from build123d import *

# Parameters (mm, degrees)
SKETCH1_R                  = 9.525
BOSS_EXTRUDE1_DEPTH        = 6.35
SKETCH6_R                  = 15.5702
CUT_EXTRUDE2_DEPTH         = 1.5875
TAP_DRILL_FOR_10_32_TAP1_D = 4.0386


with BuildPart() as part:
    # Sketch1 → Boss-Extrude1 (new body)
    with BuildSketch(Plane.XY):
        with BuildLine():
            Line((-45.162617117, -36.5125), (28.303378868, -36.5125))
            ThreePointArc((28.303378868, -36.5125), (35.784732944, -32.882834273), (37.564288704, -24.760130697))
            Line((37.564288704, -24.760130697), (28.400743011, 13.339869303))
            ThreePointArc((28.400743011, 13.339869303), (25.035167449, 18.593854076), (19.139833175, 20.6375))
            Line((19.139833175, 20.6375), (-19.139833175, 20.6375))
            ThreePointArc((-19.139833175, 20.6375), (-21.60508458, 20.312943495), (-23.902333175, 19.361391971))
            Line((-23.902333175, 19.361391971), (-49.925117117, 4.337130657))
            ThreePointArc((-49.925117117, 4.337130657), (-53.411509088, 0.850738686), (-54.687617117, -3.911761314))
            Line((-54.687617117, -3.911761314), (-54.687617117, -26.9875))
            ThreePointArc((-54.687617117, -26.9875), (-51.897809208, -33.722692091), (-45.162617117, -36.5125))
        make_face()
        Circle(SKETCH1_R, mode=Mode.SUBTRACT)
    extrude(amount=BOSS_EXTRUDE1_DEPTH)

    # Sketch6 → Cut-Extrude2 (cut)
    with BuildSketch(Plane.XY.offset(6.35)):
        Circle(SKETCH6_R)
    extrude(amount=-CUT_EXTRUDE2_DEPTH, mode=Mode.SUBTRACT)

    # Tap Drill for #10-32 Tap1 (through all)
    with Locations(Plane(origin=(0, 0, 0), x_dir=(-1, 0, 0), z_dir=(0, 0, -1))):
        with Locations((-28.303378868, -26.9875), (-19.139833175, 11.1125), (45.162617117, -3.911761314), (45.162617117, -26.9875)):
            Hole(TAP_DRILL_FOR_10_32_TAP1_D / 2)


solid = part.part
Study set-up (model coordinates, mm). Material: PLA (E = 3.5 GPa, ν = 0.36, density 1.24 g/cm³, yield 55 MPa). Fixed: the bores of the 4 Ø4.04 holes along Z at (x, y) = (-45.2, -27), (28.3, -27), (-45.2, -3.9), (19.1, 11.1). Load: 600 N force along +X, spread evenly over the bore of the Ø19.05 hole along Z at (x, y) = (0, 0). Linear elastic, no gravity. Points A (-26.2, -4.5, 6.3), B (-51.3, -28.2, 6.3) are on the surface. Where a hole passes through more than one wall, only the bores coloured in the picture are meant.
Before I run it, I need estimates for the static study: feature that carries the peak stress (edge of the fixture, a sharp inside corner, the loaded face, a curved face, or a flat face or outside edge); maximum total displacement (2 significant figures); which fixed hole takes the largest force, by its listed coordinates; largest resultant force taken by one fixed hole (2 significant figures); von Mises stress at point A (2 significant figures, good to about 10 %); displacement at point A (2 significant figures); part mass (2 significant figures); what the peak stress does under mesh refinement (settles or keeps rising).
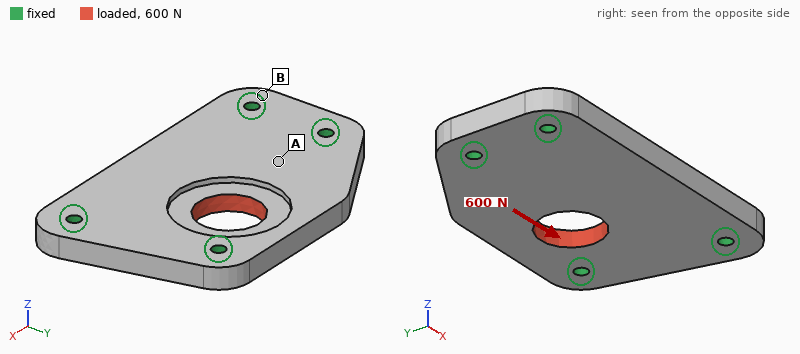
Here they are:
edge of the fixture
19 µm
(19.1, 11.1)
250 N
1.1 MPa
7.9 µm
33 g
keeps rising
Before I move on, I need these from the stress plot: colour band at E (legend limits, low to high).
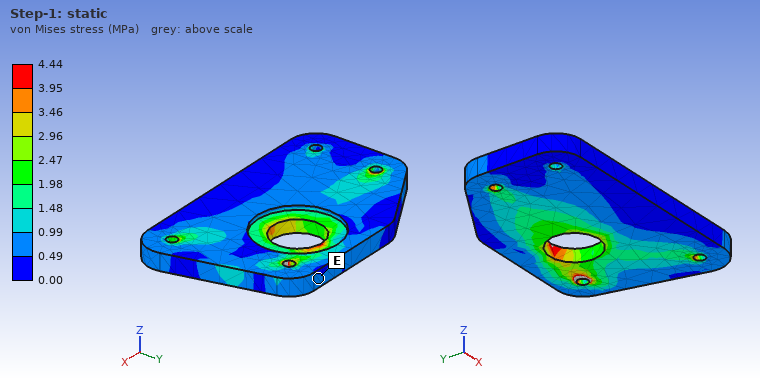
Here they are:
0.49 to 0.99 MPa
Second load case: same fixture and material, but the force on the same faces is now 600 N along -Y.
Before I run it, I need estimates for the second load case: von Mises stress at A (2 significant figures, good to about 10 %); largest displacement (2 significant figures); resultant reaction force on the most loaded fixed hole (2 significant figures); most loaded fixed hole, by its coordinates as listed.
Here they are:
1.1 MPa
42 µm
270 N
(19.1, 11.1)
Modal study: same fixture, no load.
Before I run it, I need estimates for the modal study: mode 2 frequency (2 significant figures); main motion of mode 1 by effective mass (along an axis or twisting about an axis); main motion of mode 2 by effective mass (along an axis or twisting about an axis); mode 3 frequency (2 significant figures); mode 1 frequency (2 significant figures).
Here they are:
2200 Hz
along Z
twisting about X
4200 Hz
1900 Hz
